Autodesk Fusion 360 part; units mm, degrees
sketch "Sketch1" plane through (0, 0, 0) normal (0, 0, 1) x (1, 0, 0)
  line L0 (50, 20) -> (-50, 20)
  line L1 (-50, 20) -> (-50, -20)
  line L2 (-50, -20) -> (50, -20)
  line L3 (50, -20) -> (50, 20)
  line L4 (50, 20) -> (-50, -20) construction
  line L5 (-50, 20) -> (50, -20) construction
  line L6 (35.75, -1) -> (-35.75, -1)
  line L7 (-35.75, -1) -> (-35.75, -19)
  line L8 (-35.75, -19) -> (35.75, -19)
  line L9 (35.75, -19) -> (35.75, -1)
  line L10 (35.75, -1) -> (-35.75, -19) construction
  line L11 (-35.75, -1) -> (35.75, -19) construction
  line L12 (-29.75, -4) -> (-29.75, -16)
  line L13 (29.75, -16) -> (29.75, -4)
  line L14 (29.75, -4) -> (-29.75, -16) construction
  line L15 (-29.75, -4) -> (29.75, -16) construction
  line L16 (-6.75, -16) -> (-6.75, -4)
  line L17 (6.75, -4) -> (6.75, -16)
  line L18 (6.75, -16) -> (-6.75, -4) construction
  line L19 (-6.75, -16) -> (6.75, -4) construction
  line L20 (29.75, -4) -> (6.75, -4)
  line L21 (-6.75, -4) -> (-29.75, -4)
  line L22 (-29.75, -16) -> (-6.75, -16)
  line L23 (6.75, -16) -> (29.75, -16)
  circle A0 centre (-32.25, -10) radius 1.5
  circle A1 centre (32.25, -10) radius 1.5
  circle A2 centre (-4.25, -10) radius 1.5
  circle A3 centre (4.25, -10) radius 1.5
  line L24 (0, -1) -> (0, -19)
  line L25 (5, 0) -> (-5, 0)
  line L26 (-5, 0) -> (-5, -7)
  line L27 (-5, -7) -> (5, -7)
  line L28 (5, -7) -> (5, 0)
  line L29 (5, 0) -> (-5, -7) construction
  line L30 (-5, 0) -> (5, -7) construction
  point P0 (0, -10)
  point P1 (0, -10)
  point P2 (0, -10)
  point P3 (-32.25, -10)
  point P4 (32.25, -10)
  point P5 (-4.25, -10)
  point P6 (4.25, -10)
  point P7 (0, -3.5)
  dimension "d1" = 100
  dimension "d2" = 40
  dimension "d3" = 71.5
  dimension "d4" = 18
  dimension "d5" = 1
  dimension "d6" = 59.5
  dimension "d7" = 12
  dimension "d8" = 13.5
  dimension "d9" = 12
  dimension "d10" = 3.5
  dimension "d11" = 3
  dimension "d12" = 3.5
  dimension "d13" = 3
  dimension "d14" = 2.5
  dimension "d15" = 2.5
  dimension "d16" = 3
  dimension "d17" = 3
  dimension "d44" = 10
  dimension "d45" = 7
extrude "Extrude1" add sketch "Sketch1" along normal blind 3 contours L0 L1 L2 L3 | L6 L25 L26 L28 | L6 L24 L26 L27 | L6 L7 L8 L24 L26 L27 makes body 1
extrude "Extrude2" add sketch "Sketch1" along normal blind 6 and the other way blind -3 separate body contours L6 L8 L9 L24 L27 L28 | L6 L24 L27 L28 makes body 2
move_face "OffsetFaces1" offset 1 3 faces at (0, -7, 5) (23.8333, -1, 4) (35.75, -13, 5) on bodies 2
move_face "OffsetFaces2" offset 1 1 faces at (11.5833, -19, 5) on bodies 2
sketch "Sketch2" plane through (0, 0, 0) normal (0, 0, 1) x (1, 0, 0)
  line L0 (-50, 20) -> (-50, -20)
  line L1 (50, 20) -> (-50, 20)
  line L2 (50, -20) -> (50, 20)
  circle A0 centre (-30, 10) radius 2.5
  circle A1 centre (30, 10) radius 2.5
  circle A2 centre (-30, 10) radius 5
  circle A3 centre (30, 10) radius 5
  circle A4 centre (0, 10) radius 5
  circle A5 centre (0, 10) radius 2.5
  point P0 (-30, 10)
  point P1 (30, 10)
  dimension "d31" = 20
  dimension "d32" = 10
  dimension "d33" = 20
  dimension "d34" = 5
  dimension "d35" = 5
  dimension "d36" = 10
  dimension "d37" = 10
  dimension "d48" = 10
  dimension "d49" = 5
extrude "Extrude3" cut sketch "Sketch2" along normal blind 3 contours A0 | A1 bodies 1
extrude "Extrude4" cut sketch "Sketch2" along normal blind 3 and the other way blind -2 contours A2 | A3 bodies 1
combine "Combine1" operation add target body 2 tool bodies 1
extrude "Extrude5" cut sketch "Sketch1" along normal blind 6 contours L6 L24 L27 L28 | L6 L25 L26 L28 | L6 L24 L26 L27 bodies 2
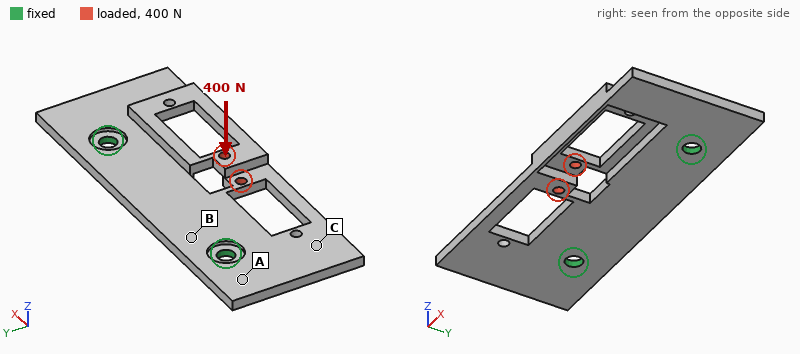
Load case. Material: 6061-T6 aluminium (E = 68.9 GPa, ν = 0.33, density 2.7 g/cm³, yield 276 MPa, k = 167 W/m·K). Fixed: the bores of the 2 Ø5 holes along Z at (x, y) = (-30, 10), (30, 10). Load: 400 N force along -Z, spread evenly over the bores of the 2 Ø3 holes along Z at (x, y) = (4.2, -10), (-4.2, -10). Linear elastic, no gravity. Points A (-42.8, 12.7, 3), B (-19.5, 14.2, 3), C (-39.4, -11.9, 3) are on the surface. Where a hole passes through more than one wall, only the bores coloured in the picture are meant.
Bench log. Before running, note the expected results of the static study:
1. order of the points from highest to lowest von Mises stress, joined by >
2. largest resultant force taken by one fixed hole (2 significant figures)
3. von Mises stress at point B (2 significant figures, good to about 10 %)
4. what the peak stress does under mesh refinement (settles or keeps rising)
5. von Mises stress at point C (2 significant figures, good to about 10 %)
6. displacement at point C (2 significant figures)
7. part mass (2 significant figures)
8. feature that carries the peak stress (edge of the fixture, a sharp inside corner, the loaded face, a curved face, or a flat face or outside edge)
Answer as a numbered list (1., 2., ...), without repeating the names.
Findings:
1. B > C > A
2. 300 N
3. 62 MPa
4. keeps rising
5. 35 MPa
6. 0.11 mm
7. 27 g
8. edge of the fixture
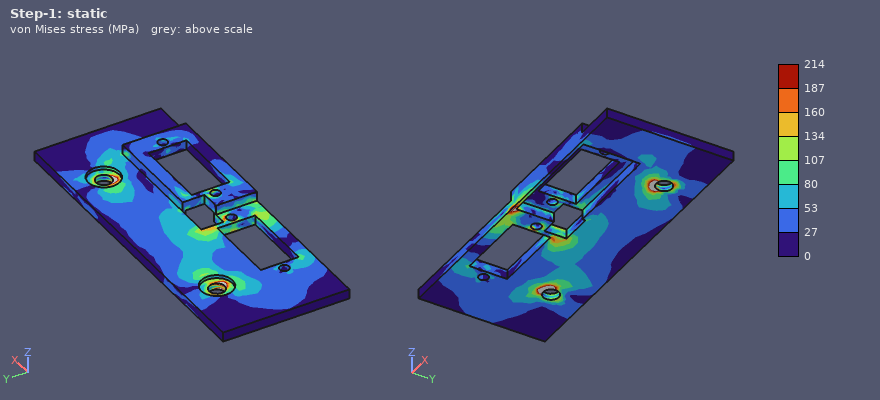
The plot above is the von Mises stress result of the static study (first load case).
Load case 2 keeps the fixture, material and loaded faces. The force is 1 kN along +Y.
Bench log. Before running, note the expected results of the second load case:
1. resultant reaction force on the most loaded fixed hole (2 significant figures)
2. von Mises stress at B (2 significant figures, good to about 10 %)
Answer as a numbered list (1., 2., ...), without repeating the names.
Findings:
1. 520 N
2. 24 MPa
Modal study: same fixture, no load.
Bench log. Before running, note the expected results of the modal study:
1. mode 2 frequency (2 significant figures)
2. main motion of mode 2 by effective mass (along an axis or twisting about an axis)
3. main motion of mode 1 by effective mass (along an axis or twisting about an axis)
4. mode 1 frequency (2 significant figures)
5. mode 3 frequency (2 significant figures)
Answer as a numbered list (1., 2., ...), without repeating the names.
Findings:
1. 2300 Hz
2. twisting about Y
3. along Z
4. 1900 Hz
5. 2800 Hz
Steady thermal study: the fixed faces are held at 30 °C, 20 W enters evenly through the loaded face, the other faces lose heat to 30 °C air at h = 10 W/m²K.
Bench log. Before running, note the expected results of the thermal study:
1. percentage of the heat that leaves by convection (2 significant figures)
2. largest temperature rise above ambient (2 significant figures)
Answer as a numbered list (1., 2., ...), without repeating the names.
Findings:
1. 6.6 %
2. 68 K
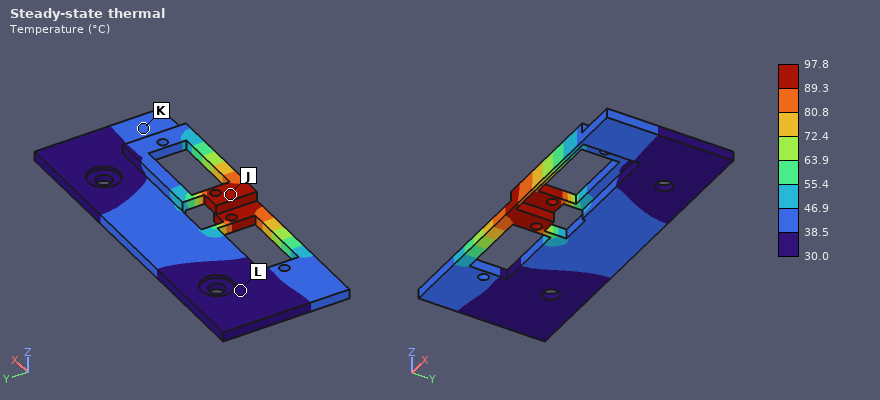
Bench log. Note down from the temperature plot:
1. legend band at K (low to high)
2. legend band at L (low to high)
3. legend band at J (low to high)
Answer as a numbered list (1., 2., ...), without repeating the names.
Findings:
1. 38.5 to 46.9 °C
2. 30.0 to 38.5 °C
3. 89.3 to 97.8 °C
